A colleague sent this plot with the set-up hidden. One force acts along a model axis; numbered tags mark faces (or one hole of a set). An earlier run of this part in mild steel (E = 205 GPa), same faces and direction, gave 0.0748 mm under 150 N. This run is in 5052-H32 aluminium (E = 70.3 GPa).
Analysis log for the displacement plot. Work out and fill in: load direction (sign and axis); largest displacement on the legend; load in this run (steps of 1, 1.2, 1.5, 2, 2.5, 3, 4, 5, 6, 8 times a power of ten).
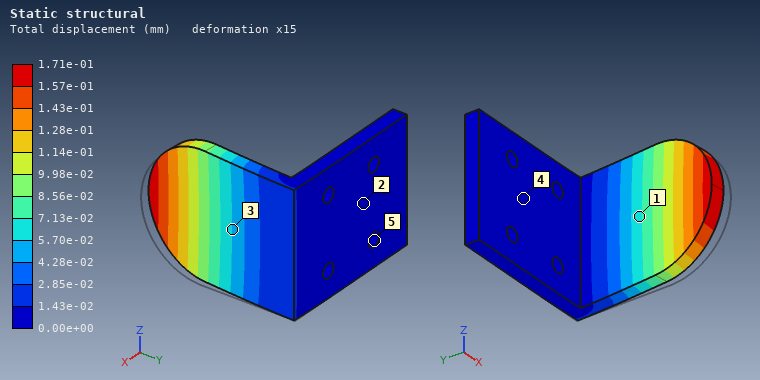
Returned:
-X
1.71e-01 mm
120 N
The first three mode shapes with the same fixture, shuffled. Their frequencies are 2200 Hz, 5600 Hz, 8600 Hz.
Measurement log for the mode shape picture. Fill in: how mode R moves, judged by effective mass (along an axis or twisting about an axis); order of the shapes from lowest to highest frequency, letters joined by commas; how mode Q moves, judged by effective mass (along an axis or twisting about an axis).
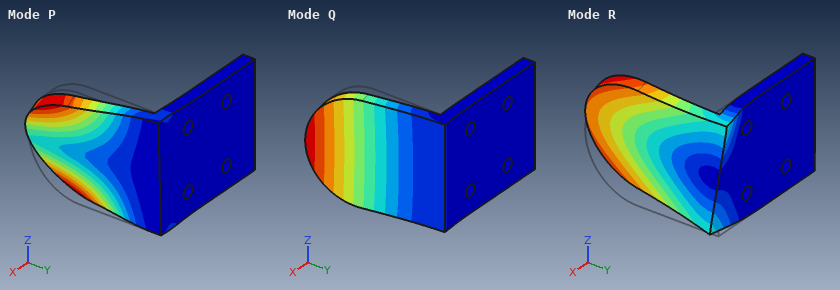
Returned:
along Z
Q, R, P
along X
